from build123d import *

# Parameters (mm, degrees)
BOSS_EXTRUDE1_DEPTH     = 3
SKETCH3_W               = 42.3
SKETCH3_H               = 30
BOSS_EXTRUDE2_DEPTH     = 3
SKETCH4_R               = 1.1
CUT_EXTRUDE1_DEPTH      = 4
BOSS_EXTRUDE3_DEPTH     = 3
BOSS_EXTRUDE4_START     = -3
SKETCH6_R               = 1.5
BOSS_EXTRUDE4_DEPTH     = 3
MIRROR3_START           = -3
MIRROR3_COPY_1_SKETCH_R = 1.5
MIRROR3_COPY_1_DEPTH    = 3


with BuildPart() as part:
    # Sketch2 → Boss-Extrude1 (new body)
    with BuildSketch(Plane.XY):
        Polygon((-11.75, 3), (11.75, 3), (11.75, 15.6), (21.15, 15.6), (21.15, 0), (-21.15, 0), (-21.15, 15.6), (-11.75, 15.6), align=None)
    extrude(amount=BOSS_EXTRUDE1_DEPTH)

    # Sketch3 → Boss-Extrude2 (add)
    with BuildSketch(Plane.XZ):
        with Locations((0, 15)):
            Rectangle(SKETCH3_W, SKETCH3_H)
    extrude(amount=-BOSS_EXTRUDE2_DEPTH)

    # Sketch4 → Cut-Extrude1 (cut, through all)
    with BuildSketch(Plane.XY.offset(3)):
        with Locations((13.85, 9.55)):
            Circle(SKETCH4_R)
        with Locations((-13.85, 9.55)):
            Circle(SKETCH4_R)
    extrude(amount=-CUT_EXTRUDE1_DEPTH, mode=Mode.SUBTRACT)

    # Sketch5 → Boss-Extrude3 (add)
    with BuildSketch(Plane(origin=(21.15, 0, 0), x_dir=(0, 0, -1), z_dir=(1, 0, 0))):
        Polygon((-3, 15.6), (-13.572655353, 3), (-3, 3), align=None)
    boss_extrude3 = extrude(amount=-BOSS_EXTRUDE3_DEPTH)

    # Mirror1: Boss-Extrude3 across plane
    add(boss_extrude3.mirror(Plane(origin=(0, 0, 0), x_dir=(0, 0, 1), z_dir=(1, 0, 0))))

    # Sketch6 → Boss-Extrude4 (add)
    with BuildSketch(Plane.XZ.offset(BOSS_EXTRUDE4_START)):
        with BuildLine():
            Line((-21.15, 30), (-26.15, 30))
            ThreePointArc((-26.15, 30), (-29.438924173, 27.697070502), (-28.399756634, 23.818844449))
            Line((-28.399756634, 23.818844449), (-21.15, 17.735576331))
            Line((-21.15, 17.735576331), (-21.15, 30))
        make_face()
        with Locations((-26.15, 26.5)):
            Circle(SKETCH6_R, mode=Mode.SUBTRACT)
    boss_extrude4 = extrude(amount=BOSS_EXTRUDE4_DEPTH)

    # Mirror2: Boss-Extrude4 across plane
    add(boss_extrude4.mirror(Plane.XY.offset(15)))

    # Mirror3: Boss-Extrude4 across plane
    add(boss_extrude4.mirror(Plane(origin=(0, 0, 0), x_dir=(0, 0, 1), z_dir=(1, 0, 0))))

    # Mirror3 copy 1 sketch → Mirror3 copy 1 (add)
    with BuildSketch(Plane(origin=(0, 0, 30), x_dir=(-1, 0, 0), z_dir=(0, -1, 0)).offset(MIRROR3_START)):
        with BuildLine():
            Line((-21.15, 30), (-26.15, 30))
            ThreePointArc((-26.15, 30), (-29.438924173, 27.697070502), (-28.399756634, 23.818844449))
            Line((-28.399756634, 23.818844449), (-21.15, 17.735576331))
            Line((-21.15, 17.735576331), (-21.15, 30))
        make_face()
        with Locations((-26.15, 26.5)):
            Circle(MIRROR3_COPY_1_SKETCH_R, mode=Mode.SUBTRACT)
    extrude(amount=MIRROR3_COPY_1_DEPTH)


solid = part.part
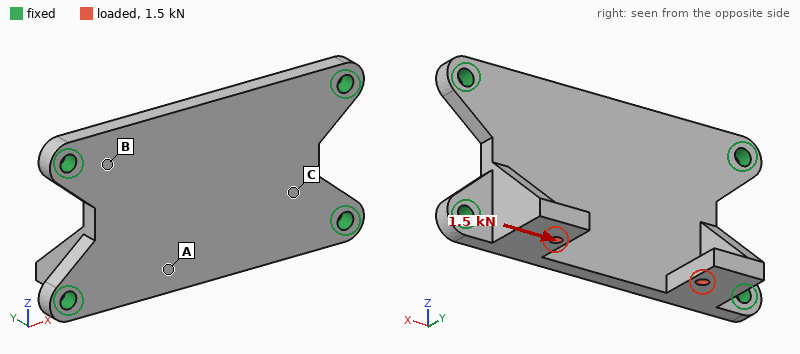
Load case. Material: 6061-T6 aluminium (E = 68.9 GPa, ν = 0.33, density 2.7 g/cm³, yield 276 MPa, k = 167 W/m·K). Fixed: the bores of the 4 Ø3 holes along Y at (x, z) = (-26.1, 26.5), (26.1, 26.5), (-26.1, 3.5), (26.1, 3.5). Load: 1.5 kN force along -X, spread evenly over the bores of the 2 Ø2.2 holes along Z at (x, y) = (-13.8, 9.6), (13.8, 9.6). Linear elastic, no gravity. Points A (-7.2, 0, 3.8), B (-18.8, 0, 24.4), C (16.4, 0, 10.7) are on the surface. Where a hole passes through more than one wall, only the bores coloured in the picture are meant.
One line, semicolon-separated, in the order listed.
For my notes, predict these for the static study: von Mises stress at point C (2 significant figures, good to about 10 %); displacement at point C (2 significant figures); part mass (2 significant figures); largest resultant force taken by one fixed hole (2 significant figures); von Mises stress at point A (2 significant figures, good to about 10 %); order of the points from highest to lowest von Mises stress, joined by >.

43 MPa; 0.017 mm; 15 g; 670 N; 75 MPa; A > C > B
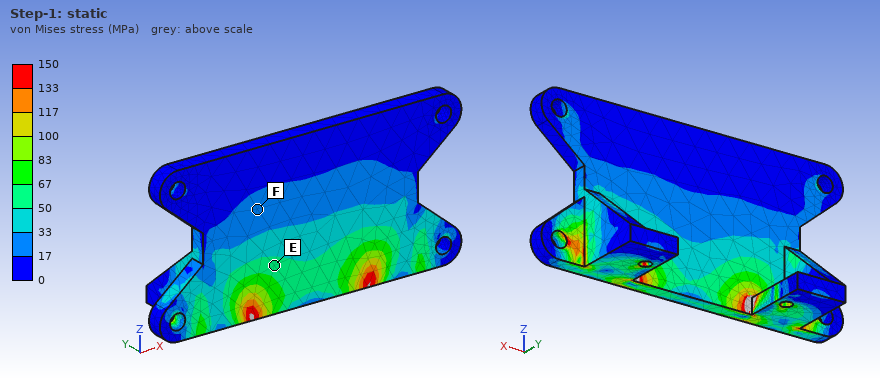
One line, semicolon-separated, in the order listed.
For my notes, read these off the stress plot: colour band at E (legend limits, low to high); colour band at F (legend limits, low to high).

50 to 67 MPa; 17 to 33 MPa
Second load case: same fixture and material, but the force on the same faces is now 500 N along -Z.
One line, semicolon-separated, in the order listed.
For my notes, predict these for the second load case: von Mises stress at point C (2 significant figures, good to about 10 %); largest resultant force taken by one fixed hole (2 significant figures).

14 MPa; 170 N
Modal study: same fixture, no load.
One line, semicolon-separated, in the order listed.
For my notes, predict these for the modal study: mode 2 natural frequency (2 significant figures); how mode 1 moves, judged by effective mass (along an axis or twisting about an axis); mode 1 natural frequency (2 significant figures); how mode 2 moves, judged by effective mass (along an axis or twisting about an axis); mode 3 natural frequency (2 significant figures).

7700 Hz; along Y; 4700 Hz; twisting about X; 11 kHz
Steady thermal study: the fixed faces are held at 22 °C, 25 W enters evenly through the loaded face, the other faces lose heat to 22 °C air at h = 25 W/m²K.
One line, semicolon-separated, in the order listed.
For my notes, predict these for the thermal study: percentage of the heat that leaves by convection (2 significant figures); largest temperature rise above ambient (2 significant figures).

4.5 %; 34 K
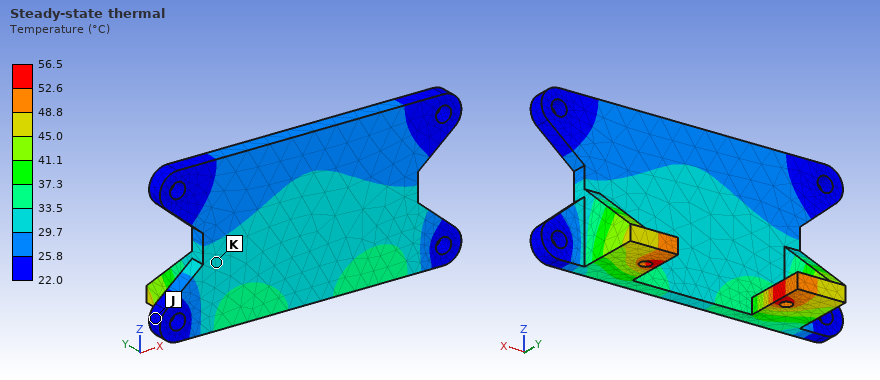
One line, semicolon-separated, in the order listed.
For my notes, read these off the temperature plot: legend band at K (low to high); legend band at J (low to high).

29.7 to 33.5 °C; 22.0 to 25.8 °C
